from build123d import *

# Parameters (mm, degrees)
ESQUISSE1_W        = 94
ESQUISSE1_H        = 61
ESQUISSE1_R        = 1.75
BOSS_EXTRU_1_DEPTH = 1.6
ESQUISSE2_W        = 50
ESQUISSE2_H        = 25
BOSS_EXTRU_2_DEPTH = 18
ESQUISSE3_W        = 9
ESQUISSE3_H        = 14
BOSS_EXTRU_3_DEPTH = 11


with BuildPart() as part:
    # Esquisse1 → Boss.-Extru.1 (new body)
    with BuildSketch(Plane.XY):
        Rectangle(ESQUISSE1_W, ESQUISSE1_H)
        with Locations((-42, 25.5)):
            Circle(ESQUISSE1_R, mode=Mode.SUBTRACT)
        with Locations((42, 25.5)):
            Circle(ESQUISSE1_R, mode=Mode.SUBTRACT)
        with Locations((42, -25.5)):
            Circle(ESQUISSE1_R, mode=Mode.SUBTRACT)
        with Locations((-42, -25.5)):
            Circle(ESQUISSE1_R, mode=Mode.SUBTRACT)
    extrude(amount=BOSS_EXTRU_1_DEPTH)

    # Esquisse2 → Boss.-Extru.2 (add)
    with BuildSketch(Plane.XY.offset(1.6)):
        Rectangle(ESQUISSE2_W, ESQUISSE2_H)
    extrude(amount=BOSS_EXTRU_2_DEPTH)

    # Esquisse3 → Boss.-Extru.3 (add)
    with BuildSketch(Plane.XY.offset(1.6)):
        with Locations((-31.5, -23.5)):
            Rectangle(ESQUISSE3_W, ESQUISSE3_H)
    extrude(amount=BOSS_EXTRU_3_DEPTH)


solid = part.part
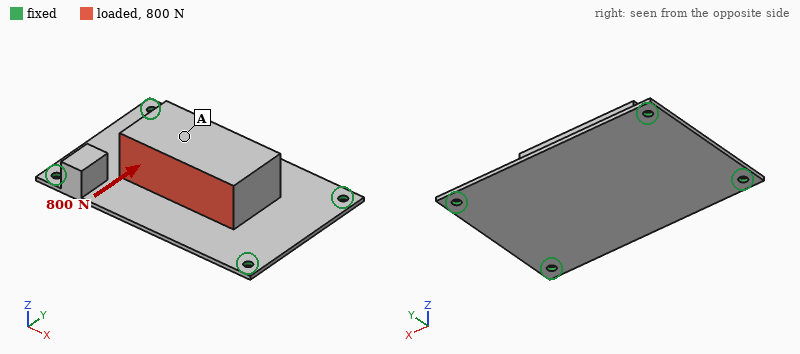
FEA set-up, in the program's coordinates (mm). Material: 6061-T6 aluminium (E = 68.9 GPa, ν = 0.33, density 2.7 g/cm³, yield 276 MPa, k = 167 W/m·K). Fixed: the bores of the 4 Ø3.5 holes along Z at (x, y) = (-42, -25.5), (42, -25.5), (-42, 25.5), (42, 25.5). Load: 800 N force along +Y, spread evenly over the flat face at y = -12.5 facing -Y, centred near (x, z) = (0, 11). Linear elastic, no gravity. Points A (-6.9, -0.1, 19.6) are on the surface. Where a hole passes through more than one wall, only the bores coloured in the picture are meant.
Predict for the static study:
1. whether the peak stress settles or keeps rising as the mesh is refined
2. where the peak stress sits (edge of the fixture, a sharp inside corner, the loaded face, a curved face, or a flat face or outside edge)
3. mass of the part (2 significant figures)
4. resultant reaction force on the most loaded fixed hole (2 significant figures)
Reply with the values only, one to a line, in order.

keeps rising
edge of the fixture
89 g
270 N
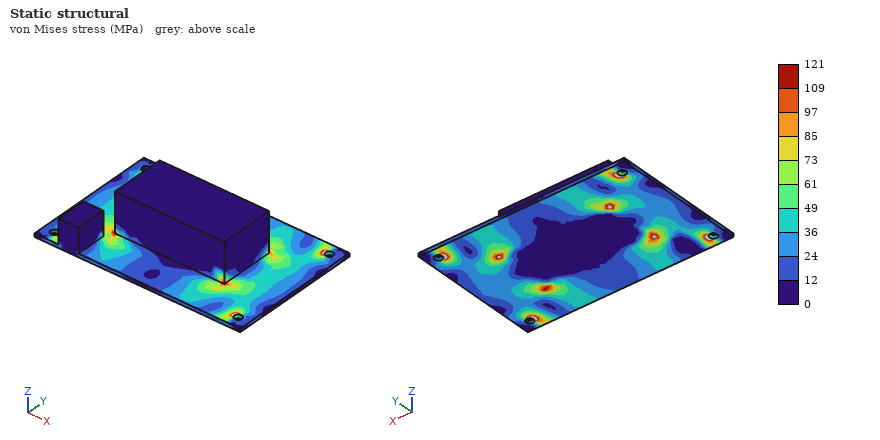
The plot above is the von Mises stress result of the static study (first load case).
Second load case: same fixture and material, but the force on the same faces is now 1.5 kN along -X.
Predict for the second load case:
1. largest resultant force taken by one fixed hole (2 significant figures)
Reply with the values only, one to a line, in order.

460 N
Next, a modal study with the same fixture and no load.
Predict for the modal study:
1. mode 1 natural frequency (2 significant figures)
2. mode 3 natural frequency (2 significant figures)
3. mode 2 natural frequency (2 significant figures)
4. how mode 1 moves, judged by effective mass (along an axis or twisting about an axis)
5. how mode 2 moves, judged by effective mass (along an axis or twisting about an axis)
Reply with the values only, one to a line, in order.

820 Hz
1600 Hz
1200 Hz
along Z
along Y
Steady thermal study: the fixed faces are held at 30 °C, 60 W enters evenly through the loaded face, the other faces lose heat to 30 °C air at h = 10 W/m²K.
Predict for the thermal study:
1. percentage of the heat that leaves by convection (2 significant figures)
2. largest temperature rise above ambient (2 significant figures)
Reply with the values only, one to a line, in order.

10 %
65 K
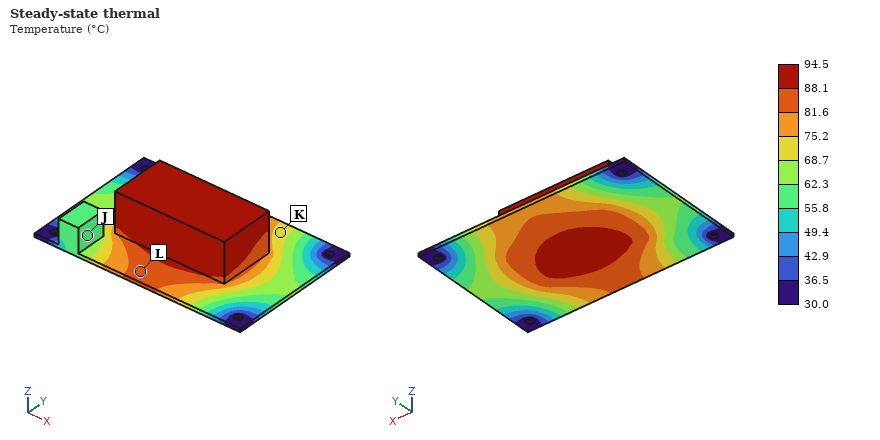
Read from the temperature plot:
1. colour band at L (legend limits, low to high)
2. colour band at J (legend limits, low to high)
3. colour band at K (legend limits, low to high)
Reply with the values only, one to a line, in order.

81.6 to 88.1 °C
55.8 to 62.3 °C
68.7 to 75.2 °C
